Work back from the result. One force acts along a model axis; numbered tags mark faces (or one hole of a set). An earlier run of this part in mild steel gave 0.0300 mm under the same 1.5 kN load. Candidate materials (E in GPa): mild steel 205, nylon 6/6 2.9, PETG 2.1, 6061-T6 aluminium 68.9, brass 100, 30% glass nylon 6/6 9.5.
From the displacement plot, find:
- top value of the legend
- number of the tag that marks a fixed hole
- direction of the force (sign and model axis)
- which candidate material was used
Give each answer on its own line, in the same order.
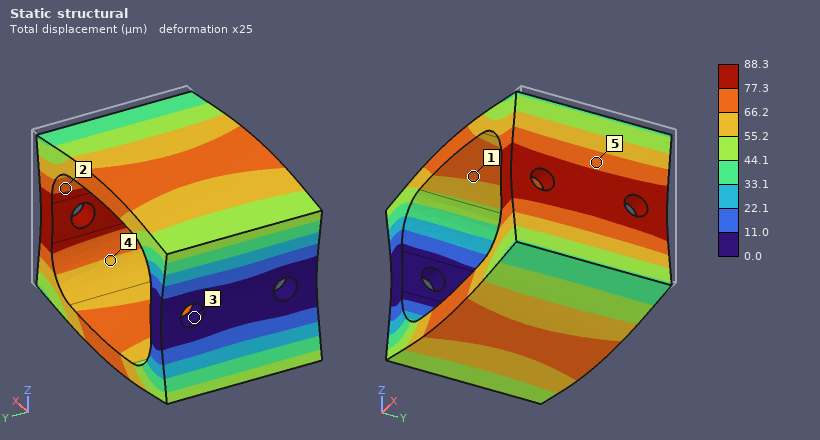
88.3 µm
3
-X
6061-T6 aluminium
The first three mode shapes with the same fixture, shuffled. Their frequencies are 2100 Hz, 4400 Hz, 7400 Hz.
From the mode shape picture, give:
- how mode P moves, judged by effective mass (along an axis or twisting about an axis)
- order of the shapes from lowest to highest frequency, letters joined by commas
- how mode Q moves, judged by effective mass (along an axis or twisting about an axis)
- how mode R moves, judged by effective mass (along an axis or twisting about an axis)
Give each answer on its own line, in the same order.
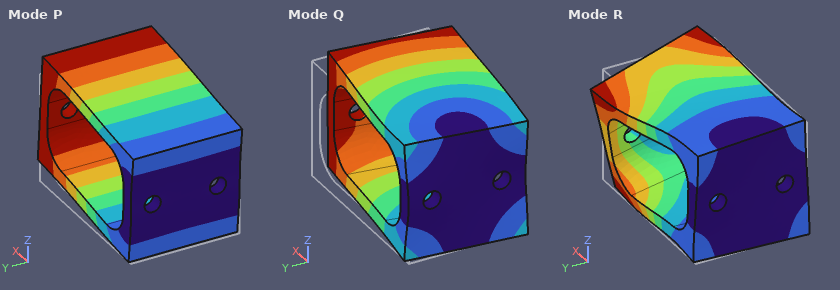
along Z
P, Q, R
along Y
twisting about X
